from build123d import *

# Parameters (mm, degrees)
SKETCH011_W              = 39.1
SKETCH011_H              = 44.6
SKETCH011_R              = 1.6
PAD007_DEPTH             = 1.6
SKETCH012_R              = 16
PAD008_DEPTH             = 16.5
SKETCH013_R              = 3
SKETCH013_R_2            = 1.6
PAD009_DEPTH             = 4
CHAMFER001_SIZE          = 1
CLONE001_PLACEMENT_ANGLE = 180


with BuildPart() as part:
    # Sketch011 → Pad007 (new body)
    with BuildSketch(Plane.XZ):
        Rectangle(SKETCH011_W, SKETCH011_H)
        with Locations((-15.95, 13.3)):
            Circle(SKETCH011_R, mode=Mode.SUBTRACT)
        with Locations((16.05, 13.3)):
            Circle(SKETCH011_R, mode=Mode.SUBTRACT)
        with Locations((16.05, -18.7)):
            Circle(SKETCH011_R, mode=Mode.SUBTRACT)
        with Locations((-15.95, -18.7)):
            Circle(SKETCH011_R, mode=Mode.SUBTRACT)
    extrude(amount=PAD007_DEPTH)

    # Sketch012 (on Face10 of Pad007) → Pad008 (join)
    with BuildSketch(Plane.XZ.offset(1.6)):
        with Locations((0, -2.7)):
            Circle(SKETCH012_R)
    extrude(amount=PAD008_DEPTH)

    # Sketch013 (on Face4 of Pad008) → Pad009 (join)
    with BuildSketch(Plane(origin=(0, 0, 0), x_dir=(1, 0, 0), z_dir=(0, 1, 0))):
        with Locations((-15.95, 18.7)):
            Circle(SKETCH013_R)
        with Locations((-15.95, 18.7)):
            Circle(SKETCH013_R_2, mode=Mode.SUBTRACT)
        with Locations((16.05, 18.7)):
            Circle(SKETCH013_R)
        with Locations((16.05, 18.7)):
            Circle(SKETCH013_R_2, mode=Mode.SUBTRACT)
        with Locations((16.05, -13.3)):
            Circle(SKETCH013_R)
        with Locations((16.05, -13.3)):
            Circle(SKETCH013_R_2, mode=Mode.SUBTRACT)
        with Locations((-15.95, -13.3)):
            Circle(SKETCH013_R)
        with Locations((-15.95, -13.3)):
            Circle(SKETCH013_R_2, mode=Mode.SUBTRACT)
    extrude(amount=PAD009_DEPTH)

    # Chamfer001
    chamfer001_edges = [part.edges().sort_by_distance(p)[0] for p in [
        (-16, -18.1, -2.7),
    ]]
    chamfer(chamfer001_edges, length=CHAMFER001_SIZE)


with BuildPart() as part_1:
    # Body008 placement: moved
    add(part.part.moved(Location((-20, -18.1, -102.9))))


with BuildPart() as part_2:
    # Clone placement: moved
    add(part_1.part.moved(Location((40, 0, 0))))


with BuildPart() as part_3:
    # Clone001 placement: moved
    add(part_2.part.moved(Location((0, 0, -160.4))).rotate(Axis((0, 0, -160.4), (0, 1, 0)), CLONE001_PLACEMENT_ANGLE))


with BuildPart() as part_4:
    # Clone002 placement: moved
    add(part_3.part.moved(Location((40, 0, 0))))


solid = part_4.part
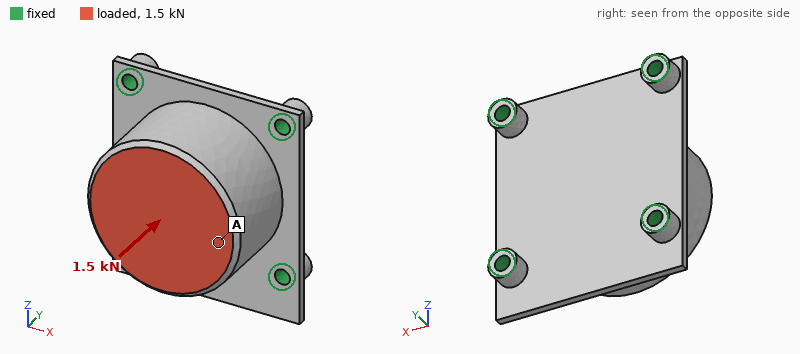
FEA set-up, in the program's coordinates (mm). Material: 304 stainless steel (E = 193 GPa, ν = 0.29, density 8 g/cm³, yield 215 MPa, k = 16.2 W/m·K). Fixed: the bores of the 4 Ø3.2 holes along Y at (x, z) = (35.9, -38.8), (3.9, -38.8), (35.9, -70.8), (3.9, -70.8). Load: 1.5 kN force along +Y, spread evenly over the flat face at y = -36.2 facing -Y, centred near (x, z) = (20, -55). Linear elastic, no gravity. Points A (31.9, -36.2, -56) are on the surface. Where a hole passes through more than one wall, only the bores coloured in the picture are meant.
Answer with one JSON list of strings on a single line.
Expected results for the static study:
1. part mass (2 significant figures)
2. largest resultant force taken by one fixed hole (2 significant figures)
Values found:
["130 g", "460 N"]
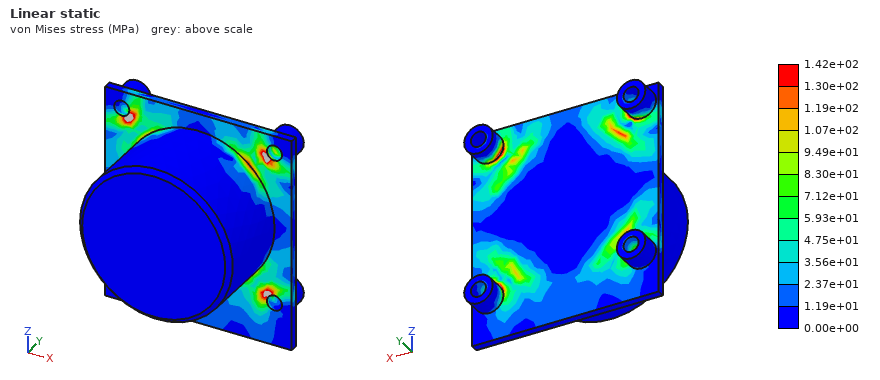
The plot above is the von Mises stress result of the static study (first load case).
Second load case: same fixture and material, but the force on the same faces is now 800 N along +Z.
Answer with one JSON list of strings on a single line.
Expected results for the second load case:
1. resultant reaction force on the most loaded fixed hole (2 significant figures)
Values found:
["360 N"]
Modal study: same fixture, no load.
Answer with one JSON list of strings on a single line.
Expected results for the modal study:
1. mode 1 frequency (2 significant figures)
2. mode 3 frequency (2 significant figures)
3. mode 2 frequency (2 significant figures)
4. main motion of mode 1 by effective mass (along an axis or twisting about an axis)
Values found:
["5500 Hz", "5800 Hz", "5700 Hz", "along Y"]
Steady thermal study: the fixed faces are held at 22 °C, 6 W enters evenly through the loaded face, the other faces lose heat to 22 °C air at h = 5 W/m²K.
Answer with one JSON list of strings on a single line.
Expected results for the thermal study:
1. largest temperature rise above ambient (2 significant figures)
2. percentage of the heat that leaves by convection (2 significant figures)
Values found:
["37 K", "9.2 %"]
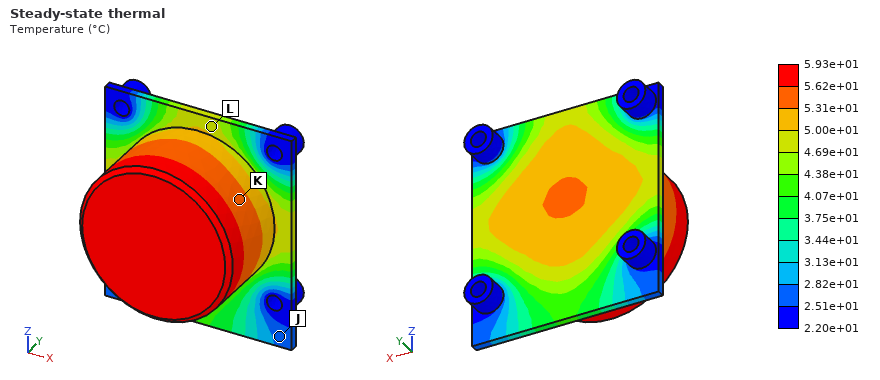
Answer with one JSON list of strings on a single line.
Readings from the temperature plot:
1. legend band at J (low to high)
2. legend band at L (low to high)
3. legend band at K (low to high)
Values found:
["2.51e+01 to 2.82e+01 °C", "4.69e+01 to 5.00e+01 °C", "5.31e+01 to 5.62e+01 °C"]
